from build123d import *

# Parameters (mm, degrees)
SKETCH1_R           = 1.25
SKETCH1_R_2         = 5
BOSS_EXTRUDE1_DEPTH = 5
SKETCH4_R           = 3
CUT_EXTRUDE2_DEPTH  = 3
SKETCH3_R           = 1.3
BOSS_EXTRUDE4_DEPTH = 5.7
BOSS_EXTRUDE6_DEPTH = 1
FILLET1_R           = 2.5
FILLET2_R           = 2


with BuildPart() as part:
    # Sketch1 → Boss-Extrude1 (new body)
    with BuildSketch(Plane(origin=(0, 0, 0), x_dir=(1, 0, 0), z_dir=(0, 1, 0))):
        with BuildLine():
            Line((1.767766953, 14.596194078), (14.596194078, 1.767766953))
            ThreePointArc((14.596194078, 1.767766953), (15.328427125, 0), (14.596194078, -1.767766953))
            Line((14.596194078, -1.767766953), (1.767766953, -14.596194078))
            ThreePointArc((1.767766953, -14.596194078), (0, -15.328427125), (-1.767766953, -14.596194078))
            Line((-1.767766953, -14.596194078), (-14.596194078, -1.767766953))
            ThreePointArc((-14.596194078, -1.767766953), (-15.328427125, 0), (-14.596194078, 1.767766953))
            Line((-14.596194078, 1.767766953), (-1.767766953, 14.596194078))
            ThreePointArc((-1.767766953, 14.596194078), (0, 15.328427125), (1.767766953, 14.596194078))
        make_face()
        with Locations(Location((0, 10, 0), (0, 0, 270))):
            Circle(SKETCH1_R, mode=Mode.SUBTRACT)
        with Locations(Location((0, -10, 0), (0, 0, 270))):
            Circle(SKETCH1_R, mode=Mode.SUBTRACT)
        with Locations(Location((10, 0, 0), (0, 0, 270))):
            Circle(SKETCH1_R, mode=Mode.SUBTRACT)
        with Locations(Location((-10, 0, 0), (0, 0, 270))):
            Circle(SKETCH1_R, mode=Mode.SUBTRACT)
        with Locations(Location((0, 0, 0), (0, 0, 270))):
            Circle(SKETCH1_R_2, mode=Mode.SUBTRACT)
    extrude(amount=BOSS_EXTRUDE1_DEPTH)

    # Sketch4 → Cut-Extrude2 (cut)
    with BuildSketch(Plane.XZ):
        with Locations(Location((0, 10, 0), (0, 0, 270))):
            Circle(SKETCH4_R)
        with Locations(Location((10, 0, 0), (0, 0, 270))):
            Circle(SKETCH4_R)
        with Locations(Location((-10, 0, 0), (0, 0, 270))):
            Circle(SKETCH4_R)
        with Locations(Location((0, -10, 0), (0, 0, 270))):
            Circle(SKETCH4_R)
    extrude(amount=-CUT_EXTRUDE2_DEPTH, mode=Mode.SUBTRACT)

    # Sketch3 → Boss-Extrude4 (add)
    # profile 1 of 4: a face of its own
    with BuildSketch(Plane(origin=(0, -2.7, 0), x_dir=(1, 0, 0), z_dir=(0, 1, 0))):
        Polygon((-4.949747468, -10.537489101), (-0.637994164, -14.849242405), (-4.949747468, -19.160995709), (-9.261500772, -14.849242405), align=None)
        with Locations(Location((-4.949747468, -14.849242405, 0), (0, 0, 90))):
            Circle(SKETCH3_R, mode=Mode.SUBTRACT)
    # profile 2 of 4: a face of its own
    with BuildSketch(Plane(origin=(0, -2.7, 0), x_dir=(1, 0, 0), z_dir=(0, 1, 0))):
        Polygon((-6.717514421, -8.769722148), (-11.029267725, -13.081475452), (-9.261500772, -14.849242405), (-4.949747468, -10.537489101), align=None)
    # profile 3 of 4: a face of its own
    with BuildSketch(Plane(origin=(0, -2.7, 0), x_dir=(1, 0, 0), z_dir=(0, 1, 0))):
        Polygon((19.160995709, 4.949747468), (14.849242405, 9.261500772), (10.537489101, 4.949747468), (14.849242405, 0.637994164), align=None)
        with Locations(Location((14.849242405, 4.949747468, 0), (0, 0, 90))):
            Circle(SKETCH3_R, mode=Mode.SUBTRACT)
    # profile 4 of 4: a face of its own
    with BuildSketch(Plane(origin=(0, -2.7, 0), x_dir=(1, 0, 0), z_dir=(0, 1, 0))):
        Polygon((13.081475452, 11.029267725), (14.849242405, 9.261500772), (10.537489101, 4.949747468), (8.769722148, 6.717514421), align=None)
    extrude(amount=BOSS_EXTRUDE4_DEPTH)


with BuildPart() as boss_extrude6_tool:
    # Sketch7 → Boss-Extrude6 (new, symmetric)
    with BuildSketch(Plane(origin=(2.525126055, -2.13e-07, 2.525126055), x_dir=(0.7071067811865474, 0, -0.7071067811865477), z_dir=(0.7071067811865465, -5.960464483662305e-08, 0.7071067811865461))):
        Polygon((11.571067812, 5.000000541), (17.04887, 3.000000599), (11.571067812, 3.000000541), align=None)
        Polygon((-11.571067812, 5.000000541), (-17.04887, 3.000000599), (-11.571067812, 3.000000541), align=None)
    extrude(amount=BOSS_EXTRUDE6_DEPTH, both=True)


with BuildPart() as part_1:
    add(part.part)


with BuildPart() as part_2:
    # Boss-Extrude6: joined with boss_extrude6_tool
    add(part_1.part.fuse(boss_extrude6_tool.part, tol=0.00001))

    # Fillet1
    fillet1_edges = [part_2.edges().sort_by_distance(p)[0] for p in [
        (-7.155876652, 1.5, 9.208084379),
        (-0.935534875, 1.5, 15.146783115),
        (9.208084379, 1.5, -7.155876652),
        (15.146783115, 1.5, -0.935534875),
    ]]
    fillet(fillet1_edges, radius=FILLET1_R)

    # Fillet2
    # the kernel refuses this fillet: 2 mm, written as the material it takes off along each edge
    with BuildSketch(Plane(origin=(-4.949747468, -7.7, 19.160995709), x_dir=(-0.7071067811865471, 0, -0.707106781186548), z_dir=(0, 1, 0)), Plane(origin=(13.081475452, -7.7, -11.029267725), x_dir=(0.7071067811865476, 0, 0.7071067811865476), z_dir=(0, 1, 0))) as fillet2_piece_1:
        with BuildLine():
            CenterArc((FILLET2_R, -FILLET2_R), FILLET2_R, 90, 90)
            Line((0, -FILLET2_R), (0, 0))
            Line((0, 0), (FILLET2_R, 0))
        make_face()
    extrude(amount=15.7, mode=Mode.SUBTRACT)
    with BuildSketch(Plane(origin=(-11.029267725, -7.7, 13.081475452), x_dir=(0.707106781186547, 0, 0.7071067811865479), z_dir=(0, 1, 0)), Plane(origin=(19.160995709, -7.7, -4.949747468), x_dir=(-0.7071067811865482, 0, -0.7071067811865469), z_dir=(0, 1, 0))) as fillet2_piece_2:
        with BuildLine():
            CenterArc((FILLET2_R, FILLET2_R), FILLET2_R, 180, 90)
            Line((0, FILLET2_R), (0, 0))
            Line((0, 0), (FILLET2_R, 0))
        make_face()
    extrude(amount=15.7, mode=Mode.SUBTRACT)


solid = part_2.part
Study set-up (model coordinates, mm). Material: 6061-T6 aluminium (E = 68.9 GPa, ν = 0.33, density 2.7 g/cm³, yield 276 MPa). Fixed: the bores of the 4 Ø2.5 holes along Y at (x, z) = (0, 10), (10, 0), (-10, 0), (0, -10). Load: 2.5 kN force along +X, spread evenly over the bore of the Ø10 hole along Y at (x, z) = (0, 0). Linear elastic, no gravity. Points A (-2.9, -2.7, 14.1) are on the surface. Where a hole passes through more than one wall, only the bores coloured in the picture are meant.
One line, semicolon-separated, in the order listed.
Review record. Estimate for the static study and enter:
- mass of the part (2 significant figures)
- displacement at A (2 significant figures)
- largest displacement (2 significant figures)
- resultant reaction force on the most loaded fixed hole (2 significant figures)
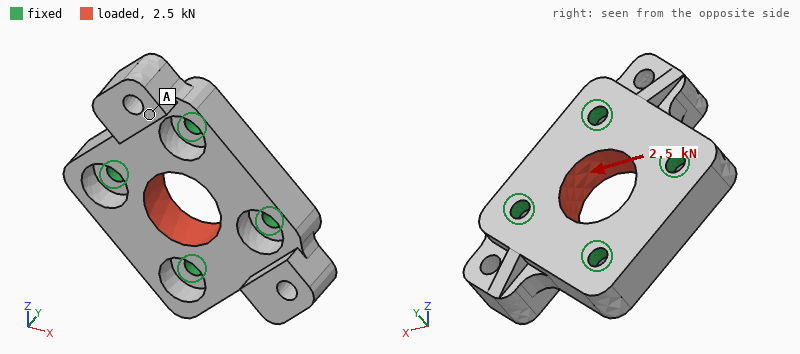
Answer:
6.5 g; 3.2 µm; 7.5 µm; 750 N
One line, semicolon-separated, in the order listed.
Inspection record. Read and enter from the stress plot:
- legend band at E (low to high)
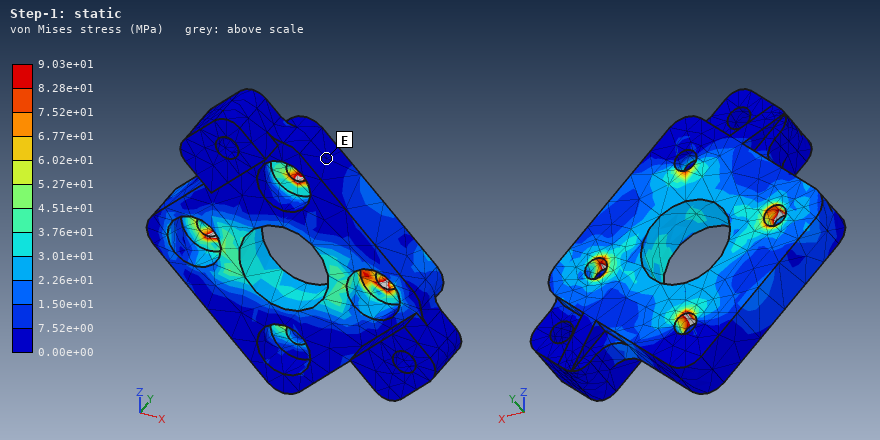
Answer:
0.00e+00 to 7.52e+00 MPa
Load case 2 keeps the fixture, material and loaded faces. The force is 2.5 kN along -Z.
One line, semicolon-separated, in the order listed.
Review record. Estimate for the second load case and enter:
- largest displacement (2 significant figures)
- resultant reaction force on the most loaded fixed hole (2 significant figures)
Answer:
7.5 µm; 750 N
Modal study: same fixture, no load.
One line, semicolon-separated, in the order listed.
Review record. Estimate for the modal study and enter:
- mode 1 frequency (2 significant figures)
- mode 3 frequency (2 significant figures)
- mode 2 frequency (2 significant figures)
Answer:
21 kHz; 41 kHz; 21 kHz
